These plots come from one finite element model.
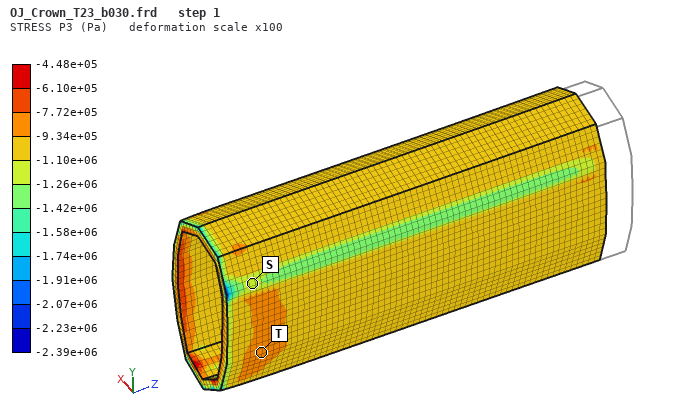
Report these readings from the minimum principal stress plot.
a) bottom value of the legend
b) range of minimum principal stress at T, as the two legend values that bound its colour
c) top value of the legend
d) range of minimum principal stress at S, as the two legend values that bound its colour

-2.39e+06 Pa
-9.34e+05 to -7.72e+05 Pa
-4.48e+05 Pa
-1.26e+06 to -1.10e+06 Pa
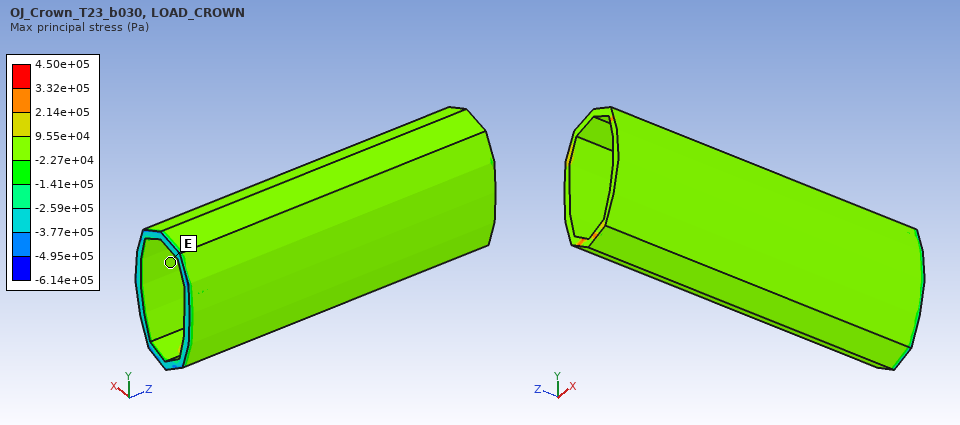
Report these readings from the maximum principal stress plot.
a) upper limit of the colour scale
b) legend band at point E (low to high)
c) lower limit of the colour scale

4.50e+05 Pa
-2.27e+04 to 9.55e+04 Pa
-6.14e+05 Pa
